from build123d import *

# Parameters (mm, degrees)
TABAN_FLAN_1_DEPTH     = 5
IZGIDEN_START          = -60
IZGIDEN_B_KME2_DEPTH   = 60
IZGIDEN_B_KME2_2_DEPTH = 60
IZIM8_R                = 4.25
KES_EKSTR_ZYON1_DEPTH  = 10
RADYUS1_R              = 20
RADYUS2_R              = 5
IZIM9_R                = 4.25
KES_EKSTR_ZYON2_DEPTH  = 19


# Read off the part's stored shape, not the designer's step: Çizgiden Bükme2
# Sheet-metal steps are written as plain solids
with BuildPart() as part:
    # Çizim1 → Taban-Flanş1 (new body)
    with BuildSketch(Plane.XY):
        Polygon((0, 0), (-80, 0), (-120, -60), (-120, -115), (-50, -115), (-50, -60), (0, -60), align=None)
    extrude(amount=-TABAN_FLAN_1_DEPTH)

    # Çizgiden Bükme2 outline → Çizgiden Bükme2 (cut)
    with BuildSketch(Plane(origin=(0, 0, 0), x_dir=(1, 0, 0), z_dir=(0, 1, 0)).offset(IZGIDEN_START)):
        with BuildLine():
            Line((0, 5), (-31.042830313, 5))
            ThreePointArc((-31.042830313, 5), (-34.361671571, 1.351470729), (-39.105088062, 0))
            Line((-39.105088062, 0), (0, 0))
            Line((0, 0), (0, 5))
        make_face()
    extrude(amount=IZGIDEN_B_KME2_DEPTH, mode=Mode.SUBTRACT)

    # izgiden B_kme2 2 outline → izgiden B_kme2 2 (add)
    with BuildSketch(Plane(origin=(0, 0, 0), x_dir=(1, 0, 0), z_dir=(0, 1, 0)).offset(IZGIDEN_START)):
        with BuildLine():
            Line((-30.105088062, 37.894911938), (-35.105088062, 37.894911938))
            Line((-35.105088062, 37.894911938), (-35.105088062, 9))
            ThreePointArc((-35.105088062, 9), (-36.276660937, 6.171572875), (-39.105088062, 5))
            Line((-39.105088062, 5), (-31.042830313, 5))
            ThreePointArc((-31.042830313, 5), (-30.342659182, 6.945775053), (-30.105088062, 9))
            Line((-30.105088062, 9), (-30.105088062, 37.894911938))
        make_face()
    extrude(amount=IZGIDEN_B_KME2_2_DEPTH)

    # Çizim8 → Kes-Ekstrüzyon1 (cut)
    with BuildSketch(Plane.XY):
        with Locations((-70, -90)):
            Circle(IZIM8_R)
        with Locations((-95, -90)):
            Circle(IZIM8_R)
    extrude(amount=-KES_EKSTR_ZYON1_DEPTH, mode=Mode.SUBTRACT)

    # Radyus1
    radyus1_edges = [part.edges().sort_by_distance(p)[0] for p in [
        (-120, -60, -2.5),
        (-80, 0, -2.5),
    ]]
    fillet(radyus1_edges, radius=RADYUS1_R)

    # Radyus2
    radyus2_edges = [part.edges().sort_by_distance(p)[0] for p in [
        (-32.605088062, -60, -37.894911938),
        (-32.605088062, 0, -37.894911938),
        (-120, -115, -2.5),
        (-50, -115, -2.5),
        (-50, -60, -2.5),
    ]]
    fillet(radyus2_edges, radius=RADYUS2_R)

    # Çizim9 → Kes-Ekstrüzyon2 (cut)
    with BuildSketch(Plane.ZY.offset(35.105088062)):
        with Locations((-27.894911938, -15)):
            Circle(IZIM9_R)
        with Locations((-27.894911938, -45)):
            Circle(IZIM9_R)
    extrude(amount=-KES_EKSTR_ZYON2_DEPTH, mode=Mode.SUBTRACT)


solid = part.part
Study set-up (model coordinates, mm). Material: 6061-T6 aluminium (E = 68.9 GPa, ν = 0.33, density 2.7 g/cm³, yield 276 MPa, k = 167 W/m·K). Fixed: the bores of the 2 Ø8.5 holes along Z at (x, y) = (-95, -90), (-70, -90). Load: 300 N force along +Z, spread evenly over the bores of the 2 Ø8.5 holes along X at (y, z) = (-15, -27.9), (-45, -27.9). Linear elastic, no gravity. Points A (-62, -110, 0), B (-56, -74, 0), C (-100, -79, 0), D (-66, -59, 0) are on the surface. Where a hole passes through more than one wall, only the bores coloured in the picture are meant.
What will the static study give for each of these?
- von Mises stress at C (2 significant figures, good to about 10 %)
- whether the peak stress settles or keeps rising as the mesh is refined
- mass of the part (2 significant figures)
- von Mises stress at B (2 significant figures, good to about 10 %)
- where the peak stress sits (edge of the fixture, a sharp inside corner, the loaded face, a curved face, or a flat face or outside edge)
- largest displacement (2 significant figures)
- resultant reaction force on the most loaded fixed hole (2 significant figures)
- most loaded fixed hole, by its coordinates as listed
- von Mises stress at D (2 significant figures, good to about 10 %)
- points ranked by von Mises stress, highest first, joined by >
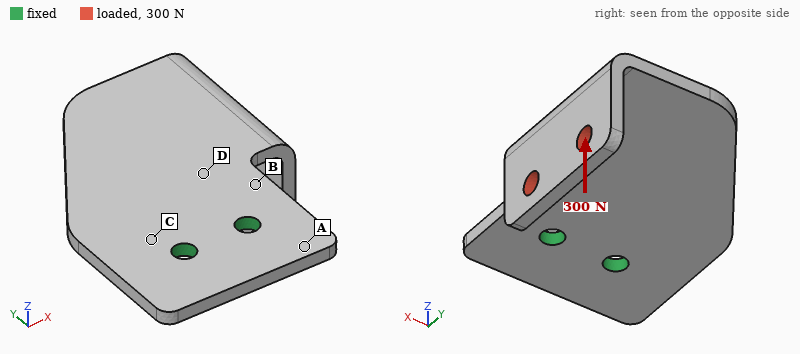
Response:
33 MPa
keeps rising
130 g
72 MPa
edge of the fixture
1.4 mm
520 N
(-70, -90)
51 MPa
B > D > C > A
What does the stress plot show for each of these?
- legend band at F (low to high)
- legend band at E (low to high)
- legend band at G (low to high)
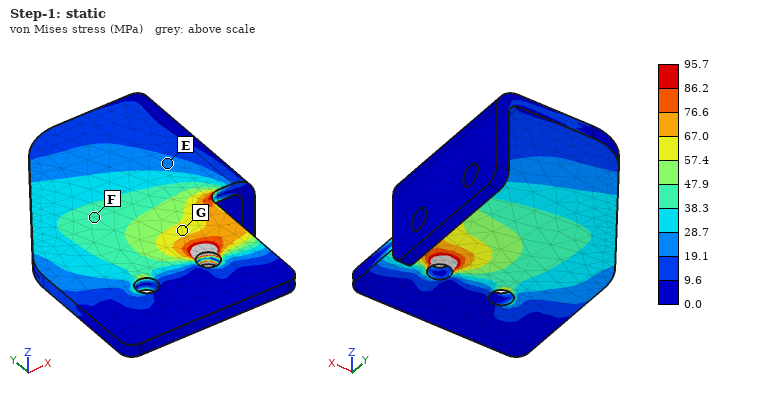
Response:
38.3 to 47.9 MPa
19.1 to 28.7 MPa
57.4 to 67.0 MPa
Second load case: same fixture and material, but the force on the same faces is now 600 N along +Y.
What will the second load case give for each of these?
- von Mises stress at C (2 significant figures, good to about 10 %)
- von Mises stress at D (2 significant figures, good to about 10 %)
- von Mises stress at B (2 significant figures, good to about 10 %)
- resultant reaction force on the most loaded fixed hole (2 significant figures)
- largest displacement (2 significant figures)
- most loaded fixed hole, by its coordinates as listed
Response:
48 MPa
58 MPa
60 MPa
1.3 kN
1.5 mm
(-70, -90)
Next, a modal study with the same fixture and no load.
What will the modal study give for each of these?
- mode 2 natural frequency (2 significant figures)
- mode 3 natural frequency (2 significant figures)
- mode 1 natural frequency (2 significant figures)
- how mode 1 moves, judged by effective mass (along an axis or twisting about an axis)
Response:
940 Hz
1800 Hz
390 Hz
along Z
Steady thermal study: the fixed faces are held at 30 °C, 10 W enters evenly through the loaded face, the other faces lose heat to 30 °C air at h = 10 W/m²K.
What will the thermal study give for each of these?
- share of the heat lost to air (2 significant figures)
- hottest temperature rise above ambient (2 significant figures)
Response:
16 %
19 K
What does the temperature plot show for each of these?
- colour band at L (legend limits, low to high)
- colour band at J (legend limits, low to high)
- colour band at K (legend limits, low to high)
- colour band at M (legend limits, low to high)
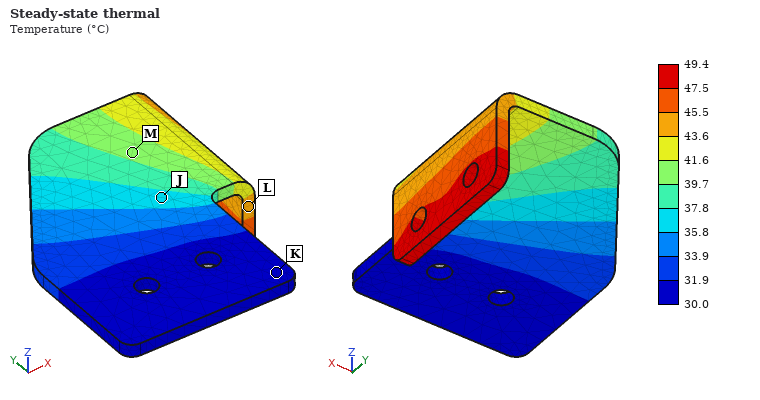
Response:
43.6 to 45.5 °C
35.8 to 37.8 °C
30.0 to 31.9 °C
39.7 to 41.6 °C
